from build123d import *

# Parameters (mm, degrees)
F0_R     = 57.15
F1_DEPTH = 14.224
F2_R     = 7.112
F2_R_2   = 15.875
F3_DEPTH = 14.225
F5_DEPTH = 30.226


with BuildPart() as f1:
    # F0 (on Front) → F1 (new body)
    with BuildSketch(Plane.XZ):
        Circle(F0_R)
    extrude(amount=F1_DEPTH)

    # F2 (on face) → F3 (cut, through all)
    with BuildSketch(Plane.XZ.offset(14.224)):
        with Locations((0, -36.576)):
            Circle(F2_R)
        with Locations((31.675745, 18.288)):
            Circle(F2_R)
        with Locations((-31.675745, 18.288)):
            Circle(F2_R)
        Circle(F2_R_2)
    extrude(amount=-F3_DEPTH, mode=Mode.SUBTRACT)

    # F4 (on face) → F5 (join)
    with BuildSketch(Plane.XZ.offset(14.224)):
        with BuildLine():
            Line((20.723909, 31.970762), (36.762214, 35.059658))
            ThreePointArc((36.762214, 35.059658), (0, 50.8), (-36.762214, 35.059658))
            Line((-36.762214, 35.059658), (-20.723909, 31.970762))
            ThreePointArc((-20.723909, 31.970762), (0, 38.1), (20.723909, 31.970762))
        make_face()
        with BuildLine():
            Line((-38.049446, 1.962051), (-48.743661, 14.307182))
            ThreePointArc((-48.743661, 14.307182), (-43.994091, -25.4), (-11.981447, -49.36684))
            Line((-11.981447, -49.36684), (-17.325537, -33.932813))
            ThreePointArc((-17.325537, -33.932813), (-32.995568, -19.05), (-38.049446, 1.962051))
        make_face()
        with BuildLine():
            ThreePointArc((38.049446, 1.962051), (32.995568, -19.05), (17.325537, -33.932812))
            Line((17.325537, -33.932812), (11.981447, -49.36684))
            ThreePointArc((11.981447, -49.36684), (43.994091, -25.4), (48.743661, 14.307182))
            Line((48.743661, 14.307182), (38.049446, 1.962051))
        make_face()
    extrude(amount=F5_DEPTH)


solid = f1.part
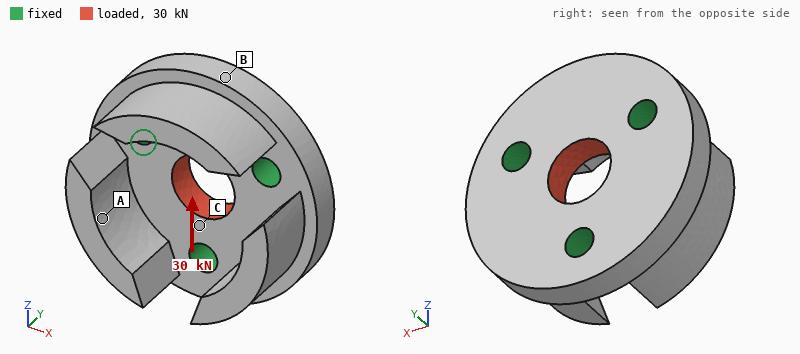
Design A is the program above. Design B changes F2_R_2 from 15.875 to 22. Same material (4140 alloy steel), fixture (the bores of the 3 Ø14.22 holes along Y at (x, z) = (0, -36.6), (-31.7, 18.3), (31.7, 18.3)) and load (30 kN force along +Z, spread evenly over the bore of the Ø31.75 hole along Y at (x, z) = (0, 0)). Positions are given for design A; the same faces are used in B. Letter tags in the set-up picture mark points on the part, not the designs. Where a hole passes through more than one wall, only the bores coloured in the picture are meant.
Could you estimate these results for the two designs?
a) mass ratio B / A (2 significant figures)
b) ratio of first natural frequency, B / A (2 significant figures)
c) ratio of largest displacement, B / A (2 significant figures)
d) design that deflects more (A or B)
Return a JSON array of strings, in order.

["0.95", "0.96", "0.84", "A"]
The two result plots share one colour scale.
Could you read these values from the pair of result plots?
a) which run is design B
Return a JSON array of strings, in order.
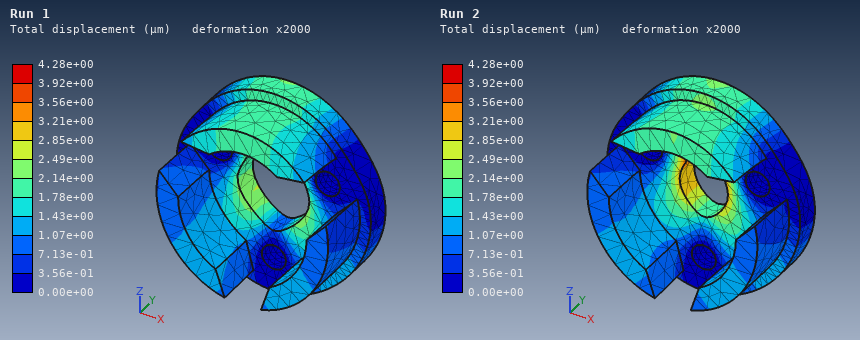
["Run 1"]
